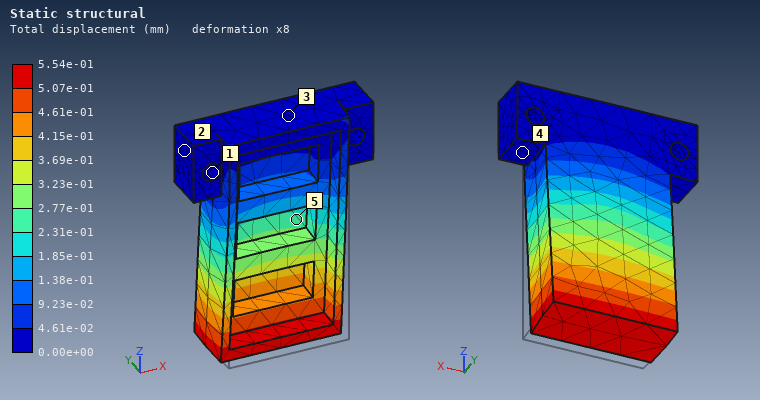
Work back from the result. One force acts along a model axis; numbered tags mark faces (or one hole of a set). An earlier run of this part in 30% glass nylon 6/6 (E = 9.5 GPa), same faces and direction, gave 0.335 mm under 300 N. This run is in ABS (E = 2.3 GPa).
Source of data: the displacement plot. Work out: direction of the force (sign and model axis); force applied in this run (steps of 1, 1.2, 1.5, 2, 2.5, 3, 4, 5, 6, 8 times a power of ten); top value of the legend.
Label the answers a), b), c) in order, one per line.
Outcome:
a) +Y
b) 120 N
c) 5.54e-01 mm
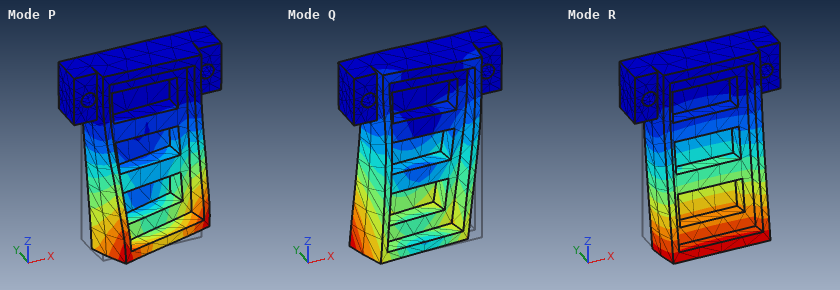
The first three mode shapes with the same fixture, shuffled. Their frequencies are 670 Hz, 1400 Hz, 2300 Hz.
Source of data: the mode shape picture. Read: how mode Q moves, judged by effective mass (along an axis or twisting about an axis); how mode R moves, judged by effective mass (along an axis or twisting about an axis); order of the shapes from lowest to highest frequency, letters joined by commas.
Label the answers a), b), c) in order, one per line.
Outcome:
a) along X
b) along Y
c) R, P, Q
